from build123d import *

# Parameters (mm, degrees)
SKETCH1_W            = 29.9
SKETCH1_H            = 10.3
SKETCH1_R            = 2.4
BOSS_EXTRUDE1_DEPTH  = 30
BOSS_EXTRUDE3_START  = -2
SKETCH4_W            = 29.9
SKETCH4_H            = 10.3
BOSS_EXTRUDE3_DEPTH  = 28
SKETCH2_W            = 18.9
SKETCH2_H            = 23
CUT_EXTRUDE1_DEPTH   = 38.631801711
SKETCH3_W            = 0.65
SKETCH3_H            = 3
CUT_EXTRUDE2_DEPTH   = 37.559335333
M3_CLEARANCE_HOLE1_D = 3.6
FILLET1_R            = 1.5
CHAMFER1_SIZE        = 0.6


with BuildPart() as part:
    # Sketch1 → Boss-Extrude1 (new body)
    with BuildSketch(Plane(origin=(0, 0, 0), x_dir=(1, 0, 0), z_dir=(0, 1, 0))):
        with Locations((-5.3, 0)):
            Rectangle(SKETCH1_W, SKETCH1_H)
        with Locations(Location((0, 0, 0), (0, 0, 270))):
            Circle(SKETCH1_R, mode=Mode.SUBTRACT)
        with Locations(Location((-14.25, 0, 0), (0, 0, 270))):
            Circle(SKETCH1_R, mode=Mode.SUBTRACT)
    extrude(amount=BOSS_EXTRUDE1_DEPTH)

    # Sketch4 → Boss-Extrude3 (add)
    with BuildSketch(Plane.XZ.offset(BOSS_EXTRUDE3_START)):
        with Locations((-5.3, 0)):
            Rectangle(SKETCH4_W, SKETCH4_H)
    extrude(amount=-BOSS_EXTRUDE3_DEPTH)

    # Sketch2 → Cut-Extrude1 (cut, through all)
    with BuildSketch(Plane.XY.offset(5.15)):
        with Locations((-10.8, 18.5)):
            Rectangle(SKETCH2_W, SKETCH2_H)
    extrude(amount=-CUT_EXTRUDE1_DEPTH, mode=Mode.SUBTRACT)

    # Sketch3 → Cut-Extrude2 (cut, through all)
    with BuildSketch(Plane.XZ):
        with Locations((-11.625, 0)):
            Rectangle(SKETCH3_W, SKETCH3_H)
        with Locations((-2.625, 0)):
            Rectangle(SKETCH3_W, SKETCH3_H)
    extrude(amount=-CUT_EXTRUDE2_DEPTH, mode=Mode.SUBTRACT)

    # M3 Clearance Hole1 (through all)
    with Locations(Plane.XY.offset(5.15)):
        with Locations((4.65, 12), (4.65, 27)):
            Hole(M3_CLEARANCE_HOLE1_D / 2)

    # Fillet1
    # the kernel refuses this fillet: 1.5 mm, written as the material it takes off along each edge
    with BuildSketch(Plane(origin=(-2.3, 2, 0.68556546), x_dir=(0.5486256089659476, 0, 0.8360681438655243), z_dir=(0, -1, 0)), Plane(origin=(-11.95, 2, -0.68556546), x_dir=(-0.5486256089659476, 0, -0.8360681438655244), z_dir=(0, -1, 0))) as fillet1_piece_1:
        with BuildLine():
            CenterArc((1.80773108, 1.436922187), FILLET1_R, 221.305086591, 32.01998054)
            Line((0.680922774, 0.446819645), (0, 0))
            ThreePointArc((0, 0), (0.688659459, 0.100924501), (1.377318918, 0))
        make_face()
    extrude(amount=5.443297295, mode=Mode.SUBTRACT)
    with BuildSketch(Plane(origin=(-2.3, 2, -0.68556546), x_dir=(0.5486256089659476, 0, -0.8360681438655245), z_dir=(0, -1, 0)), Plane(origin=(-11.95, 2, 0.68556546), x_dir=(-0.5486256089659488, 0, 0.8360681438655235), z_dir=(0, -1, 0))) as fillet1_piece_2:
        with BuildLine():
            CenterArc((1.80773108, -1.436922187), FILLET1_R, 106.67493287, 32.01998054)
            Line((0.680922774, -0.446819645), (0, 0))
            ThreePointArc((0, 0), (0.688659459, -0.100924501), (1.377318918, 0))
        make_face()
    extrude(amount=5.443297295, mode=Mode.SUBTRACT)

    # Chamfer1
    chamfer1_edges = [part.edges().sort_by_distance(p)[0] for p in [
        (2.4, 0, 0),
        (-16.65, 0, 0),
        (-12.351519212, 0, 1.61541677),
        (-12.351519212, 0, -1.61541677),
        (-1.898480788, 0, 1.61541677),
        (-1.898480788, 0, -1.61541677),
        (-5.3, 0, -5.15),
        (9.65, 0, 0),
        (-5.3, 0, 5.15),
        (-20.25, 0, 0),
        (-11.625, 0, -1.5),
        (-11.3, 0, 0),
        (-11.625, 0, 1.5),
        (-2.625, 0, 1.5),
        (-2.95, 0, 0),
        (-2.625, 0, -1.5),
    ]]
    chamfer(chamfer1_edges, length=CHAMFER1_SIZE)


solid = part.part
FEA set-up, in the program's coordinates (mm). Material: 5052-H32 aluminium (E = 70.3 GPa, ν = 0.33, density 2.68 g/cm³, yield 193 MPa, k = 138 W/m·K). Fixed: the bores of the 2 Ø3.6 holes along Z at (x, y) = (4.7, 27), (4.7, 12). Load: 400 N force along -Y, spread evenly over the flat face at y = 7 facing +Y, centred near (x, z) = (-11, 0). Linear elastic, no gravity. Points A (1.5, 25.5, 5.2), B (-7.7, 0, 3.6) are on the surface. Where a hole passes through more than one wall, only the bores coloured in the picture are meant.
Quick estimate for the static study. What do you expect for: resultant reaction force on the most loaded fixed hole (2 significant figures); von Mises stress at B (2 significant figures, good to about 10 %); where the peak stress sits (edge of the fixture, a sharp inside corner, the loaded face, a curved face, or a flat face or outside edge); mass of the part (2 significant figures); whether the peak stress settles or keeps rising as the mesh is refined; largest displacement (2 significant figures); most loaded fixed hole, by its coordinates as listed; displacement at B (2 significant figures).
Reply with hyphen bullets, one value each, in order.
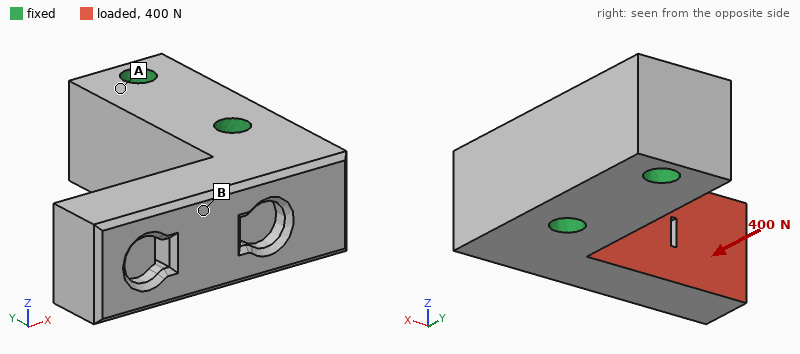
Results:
- 360 N
- 23 MPa
- a sharp inside corner
- 12 g
- keeps rising
- 63 µm
- (4.7, 12)
- 27 µm
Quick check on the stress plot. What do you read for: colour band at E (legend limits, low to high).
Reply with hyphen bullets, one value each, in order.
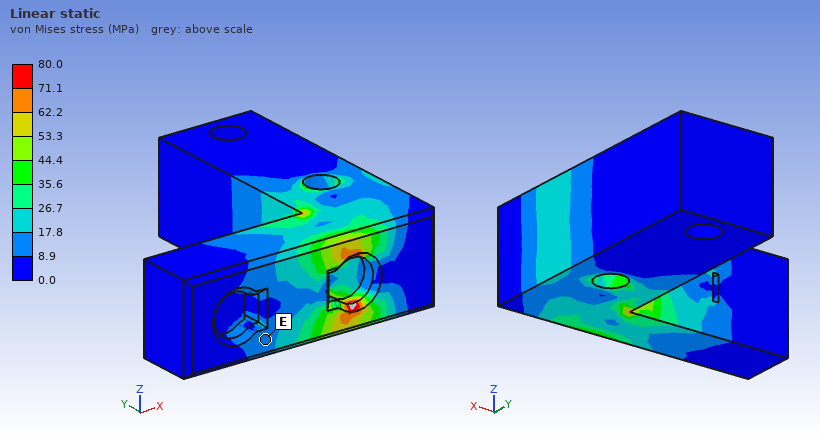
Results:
- 8.9 to 17.8 MPa
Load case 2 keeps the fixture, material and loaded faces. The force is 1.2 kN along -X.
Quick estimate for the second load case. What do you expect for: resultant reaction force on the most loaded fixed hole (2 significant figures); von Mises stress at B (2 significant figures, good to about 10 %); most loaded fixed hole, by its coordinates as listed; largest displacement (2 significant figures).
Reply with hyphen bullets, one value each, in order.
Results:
- 1.4 kN
- 25 MPa
- (4.7, 12)
- 36 µm
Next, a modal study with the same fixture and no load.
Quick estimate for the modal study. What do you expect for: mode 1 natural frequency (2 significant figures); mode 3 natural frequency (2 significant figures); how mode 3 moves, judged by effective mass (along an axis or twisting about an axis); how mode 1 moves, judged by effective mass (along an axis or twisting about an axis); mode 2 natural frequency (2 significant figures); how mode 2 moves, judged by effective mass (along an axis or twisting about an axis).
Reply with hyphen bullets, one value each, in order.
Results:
- 8300 Hz
- 26 kHz
- along X
- along Y
- 10 kHz
- along Z
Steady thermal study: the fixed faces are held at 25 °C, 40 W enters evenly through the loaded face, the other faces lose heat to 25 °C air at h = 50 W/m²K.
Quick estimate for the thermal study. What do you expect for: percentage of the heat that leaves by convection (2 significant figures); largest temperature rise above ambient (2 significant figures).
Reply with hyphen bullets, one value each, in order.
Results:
- 5.4 %
- 75 K
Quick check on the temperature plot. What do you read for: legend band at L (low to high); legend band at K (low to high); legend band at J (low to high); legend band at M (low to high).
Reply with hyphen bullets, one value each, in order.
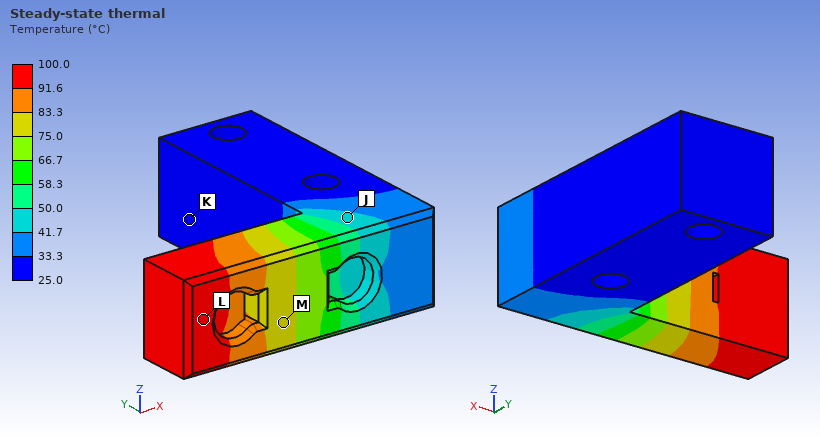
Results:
- 91.6 to 100.0 °C
- 25.0 to 33.3 °C
- 41.7 to 50.0 °C
- 75.0 to 83.3 °C
